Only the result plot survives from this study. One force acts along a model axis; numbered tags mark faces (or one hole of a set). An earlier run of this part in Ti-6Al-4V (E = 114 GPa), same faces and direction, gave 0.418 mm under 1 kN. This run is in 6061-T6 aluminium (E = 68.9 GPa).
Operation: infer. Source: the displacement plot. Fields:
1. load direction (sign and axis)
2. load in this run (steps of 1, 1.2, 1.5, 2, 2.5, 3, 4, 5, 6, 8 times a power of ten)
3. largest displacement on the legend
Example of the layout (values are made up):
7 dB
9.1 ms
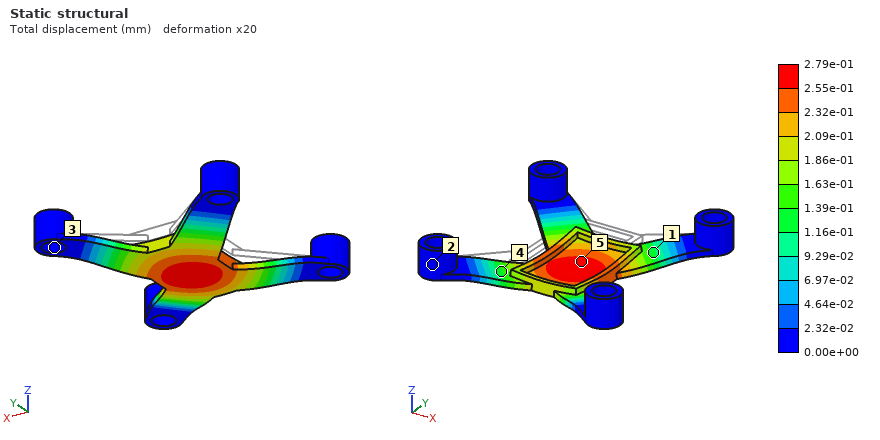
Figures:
-Z
400 N
2.79e-01 mm
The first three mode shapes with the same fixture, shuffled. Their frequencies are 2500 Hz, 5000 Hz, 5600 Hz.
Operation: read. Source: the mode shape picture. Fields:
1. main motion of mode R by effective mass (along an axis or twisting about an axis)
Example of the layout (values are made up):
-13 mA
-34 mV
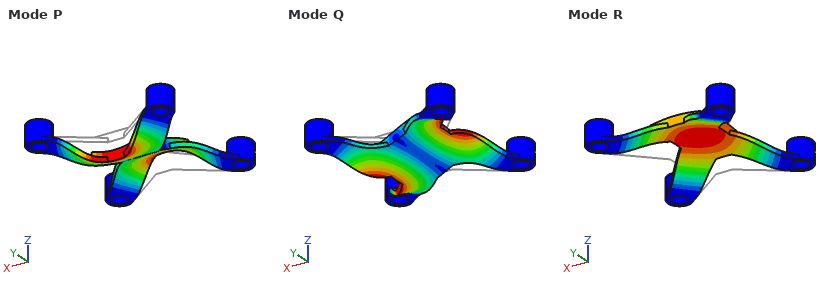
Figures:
along Z
